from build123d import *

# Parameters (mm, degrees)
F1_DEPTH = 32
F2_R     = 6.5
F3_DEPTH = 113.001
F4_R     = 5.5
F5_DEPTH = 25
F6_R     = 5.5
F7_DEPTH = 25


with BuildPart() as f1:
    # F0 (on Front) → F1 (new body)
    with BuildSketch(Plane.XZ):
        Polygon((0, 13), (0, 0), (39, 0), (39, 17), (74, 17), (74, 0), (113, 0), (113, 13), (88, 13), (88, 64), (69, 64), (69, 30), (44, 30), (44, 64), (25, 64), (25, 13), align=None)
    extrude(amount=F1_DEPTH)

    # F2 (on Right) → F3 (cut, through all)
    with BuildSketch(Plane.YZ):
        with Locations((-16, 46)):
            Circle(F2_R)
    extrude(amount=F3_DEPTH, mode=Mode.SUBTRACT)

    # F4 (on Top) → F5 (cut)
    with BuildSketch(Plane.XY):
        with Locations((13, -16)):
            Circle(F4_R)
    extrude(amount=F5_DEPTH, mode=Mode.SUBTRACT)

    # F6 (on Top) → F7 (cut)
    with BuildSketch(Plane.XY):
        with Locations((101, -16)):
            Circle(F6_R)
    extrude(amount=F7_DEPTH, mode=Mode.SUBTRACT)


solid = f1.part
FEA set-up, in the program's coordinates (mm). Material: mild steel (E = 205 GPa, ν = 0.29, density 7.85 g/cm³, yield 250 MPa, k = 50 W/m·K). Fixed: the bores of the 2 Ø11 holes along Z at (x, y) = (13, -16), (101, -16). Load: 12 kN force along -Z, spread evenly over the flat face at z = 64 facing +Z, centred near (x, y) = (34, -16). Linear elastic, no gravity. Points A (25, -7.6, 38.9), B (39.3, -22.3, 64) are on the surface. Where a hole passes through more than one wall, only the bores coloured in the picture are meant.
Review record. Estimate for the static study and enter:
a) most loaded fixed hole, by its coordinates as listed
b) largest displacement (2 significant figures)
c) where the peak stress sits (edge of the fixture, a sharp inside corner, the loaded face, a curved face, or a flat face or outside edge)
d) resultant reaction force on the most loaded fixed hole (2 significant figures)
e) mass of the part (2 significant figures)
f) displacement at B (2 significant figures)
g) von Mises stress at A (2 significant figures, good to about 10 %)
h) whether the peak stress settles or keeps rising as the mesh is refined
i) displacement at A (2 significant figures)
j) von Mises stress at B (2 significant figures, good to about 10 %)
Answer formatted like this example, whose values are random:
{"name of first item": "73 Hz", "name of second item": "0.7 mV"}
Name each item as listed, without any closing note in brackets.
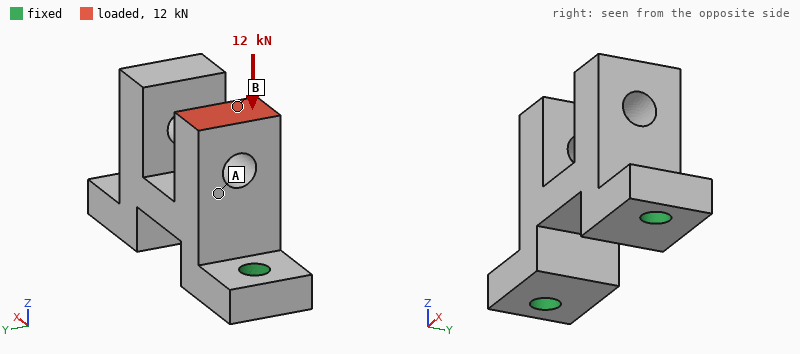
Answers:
{"most loaded fixed hole, by its coordinates as listed": "(13, -16)", "largest displacement": "17 µm", "where the peak stress sits": "edge of the fixture", "resultant reaction force on the most loaded fixed hole": "11 kN", "mass of the part": "750 g", "displacement at B": "17 µm", "von Mises stress at A": "34 MPa", "whether the peak stress settles or keeps rising as the mesh is refined": "keeps rising", "displacement at A": "13 µm", "von Mises stress at B": "17 MPa"}
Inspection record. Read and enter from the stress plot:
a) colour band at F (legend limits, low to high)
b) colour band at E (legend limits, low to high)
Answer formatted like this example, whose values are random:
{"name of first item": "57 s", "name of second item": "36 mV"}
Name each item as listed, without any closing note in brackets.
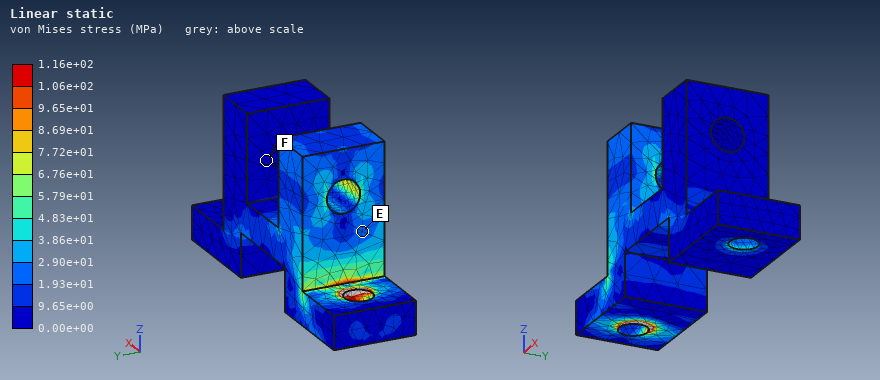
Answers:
{"colour band at F": "0.00e+00 to 9.65e+00 MPa", "colour band at E": "1.93e+01 to 2.90e+01 MPa"}
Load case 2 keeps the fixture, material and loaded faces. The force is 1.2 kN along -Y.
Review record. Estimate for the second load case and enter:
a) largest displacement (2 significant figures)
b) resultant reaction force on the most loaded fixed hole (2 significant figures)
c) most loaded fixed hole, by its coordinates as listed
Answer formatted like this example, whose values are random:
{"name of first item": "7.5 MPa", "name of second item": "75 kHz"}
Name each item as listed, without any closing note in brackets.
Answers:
{"largest displacement": "33 µm", "resultant reaction force on the most loaded fixed hole": "850 N", "most loaded fixed hole, by its coordinates as listed": "(13, -16)"}
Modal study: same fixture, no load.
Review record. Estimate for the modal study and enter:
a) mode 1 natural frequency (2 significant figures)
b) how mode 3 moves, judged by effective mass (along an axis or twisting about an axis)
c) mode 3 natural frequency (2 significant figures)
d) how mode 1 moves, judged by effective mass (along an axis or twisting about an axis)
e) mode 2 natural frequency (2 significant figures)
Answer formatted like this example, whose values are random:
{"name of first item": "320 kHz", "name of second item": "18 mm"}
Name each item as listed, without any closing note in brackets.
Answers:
{"mode 1 natural frequency": "2700 Hz", "how mode 3 moves, judged by effective mass": "along X", "mode 3 natural frequency": "5500 Hz", "how mode 1 moves, judged by effective mass": "along Y", "mode 2 natural frequency": "4500 Hz"}
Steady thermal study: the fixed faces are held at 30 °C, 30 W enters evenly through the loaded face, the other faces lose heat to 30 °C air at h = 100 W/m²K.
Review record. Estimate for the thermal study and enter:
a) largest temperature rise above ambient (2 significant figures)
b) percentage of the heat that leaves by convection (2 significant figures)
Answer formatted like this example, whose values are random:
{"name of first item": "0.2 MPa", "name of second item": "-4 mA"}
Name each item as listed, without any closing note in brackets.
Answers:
{"largest temperature rise above ambient": "49 K", "percentage of the heat that leaves by convection": "62 %"}
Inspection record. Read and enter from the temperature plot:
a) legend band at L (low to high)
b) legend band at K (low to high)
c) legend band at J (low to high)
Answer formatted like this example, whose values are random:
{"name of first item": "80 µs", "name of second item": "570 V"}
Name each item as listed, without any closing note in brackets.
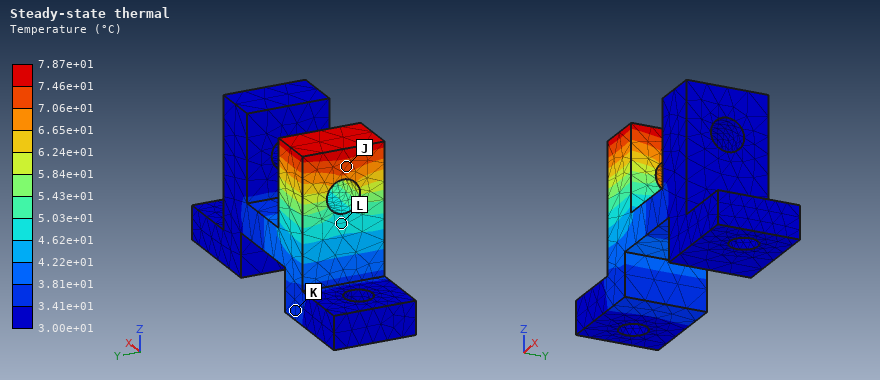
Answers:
{"legend band at L": "4.62e+01 to 5.03e+01 °C", "legend band at K": "3.41e+01 to 3.81e+01 °C", "legend band at J": "7.06e+01 to 7.46e+01 °C"}
